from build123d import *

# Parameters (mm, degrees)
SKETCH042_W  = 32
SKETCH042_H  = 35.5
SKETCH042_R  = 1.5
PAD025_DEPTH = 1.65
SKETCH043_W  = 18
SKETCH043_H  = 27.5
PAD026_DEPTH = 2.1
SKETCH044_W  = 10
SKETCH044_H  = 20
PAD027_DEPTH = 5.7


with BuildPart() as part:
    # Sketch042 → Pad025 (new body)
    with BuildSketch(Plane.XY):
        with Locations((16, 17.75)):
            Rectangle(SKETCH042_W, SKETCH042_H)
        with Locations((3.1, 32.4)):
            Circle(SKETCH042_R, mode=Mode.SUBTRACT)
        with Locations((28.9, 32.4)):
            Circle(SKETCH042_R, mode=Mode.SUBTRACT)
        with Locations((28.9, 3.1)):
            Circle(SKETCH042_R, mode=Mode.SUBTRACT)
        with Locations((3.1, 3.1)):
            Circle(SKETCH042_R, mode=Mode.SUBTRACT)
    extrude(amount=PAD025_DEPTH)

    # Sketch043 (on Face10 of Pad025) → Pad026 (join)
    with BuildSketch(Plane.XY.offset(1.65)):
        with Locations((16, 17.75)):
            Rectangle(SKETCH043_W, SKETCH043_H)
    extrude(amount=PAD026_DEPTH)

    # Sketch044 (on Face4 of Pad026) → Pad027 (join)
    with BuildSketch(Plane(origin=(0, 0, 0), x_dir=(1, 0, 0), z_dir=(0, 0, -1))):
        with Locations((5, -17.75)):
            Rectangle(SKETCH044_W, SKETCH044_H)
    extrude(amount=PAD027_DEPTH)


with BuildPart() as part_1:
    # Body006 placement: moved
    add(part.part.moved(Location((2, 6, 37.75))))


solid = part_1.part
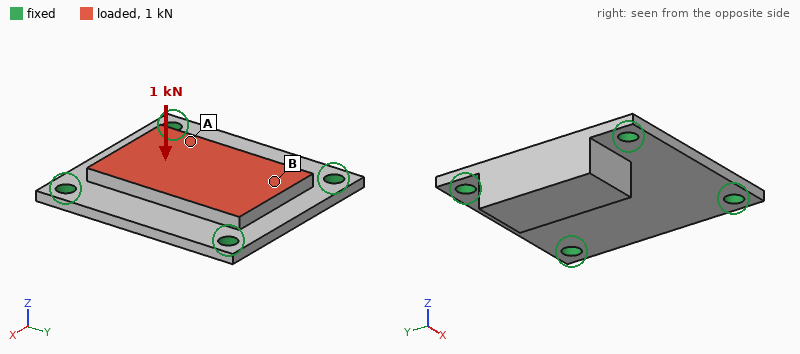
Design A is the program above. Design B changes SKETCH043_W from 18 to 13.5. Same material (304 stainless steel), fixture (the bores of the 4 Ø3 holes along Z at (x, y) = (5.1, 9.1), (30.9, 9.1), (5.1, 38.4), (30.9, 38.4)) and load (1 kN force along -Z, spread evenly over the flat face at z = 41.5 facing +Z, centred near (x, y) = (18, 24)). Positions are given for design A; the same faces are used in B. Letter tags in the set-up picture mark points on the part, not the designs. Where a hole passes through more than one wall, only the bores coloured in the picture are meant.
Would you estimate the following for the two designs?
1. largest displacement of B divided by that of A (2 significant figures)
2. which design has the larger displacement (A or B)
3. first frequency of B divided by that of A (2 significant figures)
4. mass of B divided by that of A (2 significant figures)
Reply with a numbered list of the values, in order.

1. 1.5
2. B
3. 0.88
4. 0.94
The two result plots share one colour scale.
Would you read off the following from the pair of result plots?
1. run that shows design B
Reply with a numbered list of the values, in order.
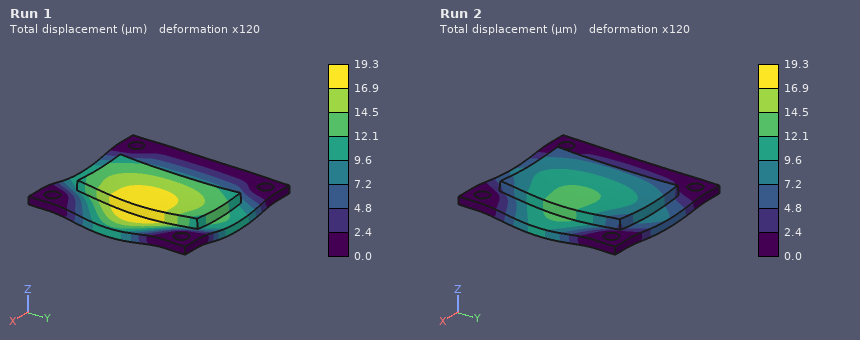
1. Run 1
